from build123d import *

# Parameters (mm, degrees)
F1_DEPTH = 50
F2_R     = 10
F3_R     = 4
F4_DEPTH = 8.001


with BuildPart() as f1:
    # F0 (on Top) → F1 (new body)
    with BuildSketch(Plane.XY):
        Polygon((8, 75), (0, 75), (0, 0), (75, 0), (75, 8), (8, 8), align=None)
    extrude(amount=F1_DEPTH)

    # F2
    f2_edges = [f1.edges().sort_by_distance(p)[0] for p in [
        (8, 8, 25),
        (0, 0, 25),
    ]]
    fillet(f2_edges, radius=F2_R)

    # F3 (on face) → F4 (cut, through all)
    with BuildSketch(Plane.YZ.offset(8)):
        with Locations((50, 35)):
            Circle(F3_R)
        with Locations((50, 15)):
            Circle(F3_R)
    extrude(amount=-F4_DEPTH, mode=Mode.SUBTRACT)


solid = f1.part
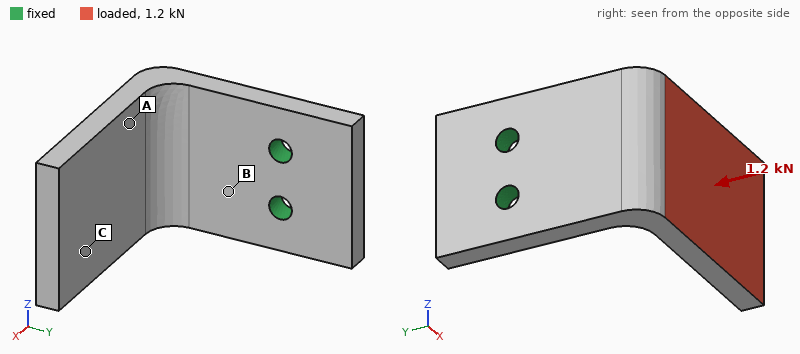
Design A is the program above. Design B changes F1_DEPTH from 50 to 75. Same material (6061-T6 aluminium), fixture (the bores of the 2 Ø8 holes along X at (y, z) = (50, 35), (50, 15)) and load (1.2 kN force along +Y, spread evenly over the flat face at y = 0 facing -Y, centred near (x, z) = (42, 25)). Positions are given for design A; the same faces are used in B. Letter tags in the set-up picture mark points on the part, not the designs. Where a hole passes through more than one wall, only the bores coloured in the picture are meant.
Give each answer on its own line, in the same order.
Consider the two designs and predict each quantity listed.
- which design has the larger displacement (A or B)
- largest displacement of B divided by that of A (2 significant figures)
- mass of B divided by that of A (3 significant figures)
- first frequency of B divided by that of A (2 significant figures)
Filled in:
A
0.72
1.51
0.94
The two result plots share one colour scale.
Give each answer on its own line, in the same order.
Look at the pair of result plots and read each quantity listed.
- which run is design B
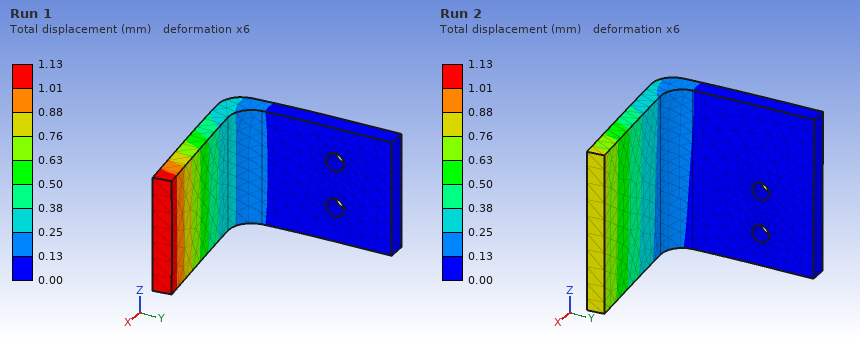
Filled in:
Run 2
